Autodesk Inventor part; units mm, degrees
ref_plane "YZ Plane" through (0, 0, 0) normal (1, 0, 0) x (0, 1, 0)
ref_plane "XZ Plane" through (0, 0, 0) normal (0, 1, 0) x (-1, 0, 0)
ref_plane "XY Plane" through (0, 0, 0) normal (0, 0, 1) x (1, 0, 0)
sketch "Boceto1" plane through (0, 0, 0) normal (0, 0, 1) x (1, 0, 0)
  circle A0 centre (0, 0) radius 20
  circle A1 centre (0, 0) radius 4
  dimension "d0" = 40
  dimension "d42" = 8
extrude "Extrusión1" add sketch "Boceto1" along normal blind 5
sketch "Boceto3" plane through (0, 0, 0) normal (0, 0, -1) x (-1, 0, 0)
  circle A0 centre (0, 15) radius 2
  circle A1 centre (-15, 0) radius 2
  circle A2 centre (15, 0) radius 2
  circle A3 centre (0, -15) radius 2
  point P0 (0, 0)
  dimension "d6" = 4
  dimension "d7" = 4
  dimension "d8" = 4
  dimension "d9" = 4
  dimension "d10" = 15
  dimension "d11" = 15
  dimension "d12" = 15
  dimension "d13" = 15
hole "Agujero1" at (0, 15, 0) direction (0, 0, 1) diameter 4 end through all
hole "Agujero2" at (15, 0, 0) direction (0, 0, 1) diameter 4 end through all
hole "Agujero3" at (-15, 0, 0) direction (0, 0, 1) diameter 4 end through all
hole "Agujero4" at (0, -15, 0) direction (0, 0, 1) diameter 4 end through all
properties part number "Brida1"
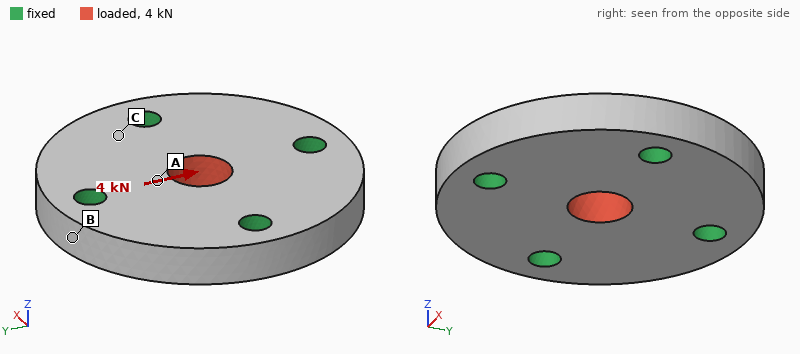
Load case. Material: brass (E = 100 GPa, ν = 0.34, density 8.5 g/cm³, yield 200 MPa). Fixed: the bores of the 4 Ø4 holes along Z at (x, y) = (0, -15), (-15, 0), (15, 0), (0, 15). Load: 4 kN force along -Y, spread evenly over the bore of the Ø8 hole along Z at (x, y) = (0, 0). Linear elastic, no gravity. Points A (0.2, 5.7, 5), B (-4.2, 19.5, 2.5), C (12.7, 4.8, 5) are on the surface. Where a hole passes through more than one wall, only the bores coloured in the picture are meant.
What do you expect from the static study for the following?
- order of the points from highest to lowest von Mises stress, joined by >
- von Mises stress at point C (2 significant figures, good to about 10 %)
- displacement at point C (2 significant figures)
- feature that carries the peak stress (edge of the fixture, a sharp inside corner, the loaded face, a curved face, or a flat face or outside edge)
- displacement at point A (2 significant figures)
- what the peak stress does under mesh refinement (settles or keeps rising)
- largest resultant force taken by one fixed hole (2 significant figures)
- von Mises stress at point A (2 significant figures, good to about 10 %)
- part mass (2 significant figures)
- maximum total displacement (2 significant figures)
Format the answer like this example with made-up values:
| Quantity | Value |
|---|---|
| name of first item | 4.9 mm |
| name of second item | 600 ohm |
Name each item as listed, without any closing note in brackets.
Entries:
| Quantity | Value |
|---|---|
| order of the points from highest to lowest von Mises stress, joined by > | A > C > B |
| von Mises stress at point C | 10 MPa |
| displacement at point C | 0.78 µm |
| feature that carries the peak stress | edge of the fixture |
| displacement at point A | 2.6 µm |
| what the peak stress does under mesh refinement | keeps rising |
| largest resultant force taken by one fixed hole | 1.3 kN |
| von Mises stress at point A | 35 MPa |
| part mass | 49 g |
| maximum total displacement | 3.6 µm |
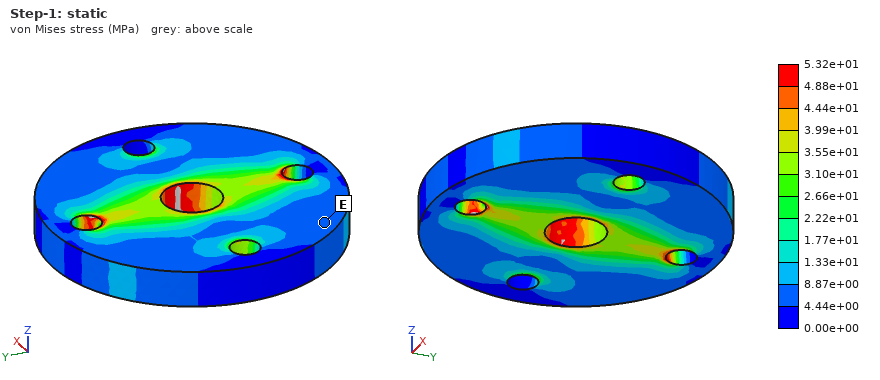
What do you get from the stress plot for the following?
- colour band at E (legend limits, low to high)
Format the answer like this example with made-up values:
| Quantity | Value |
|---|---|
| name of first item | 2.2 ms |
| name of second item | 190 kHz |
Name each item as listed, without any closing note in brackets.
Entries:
| Quantity | Value |
|---|---|
| colour band at E | 4.44e+00 to 8.87e+00 MPa |
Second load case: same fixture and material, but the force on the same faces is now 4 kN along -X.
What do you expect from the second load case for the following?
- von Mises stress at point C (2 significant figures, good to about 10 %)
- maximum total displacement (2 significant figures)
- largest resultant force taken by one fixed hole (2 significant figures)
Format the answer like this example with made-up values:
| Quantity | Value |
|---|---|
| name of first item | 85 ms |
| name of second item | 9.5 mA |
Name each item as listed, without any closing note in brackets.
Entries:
| Quantity | Value |
|---|---|
| von Mises stress at point C | 12 MPa |
| maximum total displacement | 3.6 µm |
| largest resultant force taken by one fixed hole | 1.3 kN |
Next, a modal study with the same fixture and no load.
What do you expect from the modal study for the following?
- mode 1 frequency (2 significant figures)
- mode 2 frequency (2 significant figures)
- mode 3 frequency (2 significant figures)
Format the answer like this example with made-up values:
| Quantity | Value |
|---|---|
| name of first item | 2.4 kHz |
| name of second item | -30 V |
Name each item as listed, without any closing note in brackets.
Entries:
| Quantity | Value |
|---|---|
| mode 1 frequency | 24 kHz |
| mode 2 frequency | 25 kHz |
| mode 3 frequency | 25 kHz |
